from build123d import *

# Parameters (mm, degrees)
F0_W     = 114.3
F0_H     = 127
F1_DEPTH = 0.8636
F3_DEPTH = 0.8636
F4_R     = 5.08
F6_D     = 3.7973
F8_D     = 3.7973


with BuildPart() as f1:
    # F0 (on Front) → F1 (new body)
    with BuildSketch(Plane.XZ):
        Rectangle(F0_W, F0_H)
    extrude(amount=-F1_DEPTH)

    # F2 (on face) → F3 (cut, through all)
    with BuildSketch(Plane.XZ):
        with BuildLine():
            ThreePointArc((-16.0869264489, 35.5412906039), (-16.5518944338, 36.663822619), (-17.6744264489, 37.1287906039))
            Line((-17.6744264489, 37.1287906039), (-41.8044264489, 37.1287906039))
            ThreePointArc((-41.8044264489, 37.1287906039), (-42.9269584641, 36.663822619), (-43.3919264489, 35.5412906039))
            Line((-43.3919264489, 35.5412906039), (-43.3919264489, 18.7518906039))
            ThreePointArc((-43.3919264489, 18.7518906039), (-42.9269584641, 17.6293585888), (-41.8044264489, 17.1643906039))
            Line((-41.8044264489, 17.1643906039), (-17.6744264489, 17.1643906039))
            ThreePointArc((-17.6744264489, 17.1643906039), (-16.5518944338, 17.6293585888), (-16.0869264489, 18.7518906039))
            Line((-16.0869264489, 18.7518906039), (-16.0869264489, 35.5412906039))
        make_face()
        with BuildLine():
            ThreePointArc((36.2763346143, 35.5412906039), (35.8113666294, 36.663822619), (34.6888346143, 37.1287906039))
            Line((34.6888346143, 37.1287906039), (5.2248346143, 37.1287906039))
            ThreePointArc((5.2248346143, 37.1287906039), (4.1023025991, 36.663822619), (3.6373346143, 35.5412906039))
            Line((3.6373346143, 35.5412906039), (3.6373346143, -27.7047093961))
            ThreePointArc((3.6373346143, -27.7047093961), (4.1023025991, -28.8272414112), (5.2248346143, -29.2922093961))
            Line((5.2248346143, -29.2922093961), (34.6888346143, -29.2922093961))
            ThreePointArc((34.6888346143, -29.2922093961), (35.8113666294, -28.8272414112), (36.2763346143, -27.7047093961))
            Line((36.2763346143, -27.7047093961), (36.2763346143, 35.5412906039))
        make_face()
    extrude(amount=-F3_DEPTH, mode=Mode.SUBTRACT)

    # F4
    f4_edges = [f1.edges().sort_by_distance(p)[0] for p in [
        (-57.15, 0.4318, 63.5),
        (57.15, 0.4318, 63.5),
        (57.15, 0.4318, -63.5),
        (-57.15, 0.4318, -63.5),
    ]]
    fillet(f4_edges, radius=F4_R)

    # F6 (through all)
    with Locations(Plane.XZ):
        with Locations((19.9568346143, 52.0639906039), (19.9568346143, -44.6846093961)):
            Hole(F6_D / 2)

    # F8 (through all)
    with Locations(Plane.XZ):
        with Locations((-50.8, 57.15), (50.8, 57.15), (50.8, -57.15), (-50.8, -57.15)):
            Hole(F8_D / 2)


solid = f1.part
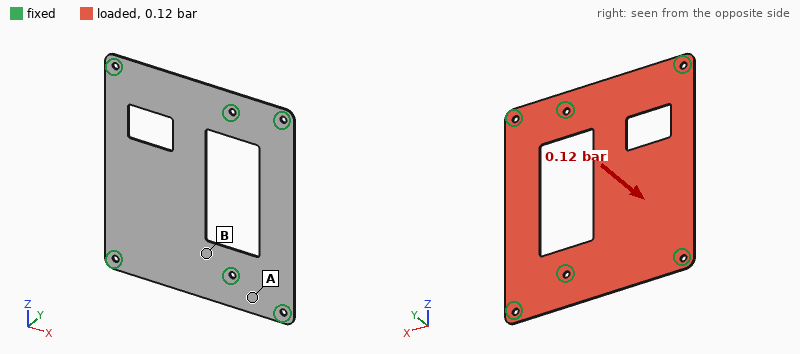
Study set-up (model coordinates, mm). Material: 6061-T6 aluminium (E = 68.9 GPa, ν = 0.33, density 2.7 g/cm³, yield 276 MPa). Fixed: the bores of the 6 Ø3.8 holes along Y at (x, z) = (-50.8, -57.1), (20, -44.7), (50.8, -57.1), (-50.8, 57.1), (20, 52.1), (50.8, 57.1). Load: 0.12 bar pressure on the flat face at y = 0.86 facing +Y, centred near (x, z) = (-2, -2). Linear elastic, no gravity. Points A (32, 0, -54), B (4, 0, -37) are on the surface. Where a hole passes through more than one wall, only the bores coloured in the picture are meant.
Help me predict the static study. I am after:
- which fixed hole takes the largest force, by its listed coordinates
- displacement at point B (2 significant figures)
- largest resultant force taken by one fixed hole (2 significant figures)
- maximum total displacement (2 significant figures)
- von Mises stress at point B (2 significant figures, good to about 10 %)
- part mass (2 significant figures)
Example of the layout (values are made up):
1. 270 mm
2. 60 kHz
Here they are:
1. (20, -44.7)
2. 0.34 mm
3. 38 N
4. 1.7 mm
5. 32 MPa
6. 27 g
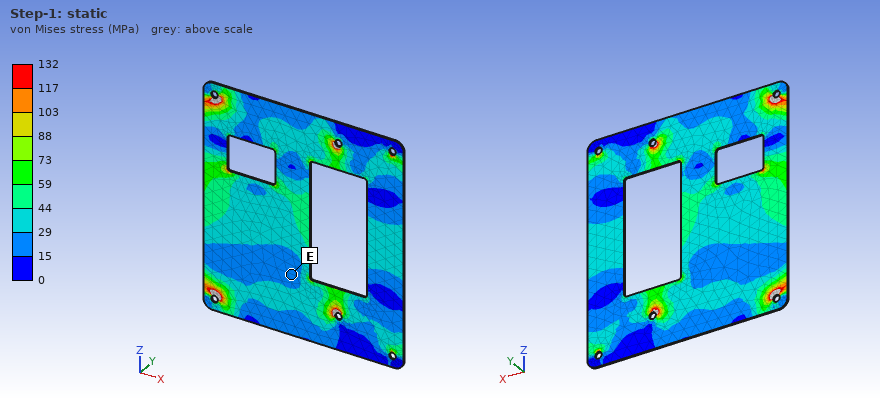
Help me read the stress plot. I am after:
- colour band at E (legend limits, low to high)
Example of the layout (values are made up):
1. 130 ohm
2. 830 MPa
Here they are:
1. 15 to 29 MPa
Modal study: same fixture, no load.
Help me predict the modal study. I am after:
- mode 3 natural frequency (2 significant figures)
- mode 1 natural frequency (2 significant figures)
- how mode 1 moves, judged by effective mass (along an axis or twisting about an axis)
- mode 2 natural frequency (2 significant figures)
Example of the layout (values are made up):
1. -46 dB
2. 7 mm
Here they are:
1. 600 Hz
2. 330 Hz
3. along Y
4. 440 Hz
